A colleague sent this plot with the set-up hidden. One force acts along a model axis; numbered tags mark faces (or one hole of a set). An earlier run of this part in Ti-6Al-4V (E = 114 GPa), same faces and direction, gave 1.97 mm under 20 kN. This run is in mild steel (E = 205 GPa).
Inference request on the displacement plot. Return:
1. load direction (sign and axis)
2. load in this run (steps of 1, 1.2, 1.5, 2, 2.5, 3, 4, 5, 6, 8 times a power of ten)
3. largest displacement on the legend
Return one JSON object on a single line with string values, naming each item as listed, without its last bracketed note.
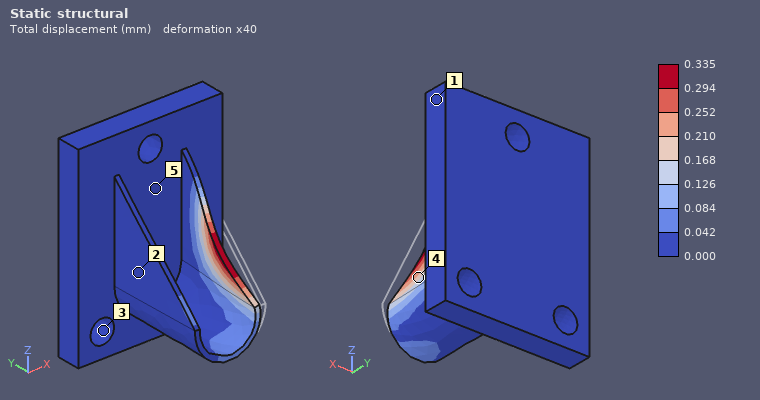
{"load direction": "-X", "load in this run": "6 kN", "largest displacement on the legend": "0.335 mm"}
